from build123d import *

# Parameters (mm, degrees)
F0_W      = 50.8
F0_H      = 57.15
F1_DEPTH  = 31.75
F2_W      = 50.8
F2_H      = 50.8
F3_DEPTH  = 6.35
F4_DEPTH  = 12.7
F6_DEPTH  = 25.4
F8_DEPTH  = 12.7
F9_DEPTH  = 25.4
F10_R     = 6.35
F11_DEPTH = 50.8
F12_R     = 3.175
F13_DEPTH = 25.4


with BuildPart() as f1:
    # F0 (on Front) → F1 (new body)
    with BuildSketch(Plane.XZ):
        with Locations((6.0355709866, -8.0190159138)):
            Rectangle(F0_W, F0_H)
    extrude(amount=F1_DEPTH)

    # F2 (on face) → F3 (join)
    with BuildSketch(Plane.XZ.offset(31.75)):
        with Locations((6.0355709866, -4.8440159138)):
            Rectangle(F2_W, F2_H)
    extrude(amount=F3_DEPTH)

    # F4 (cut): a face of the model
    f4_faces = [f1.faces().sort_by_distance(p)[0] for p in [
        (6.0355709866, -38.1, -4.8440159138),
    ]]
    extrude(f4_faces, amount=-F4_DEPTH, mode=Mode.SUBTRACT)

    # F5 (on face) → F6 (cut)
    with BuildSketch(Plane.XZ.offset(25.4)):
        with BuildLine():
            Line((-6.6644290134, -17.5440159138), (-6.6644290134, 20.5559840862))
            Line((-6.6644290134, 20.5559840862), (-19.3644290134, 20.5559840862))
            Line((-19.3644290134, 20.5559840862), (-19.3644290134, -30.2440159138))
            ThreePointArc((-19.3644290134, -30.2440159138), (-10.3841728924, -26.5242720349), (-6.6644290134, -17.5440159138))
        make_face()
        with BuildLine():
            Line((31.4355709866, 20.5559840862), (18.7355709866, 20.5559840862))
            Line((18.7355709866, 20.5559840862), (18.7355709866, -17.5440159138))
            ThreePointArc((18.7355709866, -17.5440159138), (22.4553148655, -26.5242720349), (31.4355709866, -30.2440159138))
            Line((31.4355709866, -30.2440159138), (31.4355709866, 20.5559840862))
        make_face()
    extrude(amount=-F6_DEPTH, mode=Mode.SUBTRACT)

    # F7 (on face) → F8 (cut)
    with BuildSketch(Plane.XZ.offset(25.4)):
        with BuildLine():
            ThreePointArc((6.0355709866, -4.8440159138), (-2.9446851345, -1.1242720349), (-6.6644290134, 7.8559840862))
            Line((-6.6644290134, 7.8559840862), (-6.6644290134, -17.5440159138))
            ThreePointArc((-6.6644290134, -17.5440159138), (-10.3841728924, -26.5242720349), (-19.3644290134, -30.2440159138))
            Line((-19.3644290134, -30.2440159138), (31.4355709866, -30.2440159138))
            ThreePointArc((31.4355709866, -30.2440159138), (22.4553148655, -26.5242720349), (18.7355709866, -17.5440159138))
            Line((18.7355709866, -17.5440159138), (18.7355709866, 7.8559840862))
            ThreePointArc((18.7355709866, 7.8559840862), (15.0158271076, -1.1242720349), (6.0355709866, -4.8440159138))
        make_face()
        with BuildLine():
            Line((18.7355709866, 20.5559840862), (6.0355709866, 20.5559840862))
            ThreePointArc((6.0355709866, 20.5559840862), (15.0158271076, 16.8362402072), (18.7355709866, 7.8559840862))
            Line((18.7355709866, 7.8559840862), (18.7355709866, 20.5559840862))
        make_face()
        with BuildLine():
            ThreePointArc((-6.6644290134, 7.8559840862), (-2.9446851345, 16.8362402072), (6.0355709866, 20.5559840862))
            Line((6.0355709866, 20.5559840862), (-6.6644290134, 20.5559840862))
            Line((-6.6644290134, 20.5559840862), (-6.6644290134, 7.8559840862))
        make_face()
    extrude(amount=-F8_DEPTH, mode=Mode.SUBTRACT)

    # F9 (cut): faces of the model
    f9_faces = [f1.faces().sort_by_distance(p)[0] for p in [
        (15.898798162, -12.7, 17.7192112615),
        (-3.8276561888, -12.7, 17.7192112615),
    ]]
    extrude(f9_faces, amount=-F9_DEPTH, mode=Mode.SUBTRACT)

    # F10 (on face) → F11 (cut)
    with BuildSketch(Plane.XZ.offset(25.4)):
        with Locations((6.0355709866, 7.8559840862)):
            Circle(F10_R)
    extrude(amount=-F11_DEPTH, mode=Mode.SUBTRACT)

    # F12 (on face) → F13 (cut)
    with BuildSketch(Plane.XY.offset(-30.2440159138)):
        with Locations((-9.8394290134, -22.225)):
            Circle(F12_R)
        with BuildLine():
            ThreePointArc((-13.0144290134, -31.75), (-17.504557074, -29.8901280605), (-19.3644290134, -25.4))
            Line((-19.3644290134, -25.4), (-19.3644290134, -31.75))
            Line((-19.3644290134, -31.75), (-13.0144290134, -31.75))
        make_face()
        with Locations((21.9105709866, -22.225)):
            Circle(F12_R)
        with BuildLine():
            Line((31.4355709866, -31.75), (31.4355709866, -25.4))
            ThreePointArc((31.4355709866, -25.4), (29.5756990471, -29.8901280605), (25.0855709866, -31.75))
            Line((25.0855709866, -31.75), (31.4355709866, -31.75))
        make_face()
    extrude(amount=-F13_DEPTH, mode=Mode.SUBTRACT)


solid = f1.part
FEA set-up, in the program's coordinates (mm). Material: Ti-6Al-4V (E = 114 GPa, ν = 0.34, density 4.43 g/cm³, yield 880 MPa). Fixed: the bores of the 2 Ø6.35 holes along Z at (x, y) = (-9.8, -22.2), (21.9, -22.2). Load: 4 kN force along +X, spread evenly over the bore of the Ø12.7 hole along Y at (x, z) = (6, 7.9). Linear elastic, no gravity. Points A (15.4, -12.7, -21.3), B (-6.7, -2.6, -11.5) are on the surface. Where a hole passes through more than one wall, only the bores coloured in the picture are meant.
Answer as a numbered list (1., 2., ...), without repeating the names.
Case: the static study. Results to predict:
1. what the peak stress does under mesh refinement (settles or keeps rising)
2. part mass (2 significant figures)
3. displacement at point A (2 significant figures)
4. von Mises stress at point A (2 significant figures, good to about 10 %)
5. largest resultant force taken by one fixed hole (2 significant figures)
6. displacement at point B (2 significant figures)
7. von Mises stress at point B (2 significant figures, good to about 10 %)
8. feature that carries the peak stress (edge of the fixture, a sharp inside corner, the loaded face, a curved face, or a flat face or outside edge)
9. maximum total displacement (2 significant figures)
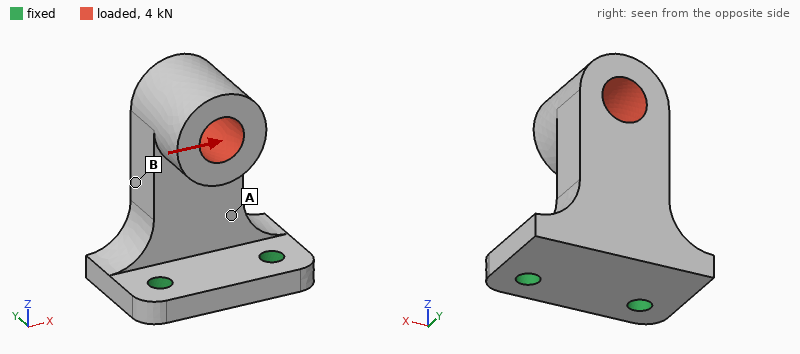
1. keeps rising
2. 130 g
3. 0.046 mm
4. 110 MPa
5. 5.4 kN
6. 0.078 mm
7. 54 MPa
8. edge of the fixture
9. 0.24 mm
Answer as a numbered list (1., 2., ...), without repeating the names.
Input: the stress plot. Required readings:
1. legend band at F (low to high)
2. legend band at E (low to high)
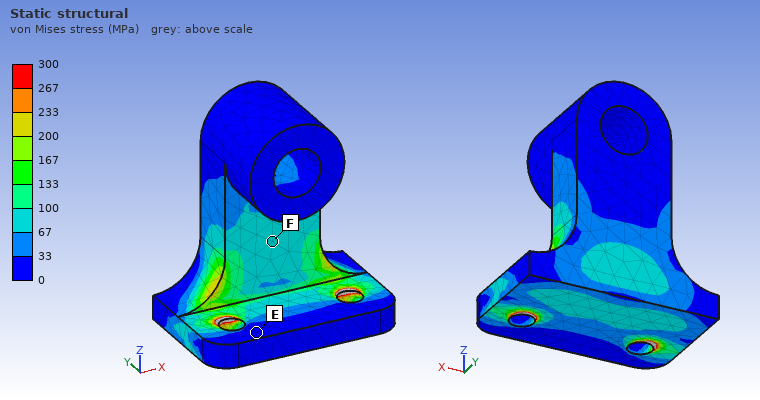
1. 67 to 100 MPa
2. 0 to 33 MPa
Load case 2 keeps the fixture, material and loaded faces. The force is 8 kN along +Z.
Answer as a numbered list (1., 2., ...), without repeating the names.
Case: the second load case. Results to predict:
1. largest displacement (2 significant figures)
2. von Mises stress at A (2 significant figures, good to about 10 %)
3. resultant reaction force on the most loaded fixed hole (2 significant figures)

1. 81 µm
2. 94 MPa
3. 4.0 kN
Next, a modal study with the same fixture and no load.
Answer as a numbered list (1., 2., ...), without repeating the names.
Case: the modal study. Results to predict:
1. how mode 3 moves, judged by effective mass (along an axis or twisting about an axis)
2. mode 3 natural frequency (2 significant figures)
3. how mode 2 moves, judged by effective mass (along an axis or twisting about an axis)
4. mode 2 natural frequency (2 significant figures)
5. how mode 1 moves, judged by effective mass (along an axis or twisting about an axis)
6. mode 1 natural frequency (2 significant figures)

1. along Z
2. 6500 Hz
3. along X
4. 3400 Hz
5. along Y
6. 1500 Hz
